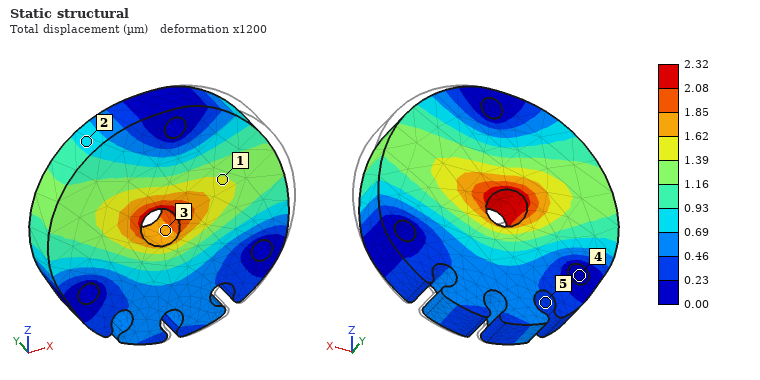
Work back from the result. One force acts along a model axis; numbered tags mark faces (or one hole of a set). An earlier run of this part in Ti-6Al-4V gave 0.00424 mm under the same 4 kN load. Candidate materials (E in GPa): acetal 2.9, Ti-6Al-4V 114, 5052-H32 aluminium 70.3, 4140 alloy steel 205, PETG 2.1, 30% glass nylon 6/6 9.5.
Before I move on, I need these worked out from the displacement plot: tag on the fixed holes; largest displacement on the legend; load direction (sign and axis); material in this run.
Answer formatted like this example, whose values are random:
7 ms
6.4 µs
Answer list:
4
2.32 µm
-X
4140 alloy steel
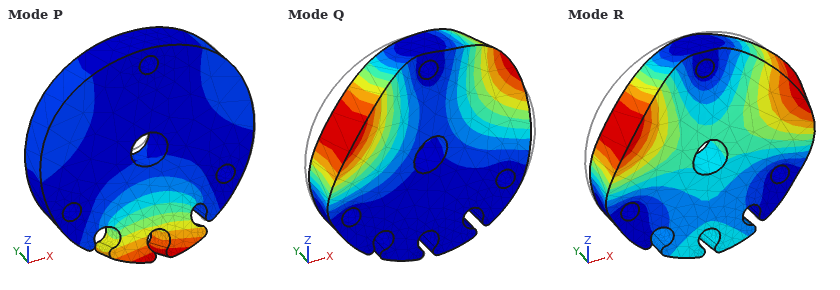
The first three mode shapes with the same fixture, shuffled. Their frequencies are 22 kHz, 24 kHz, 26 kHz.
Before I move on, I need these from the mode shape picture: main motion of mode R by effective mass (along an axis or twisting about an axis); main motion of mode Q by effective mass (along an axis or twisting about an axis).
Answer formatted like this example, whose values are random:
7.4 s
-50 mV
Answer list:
along Y
twisting about Z
